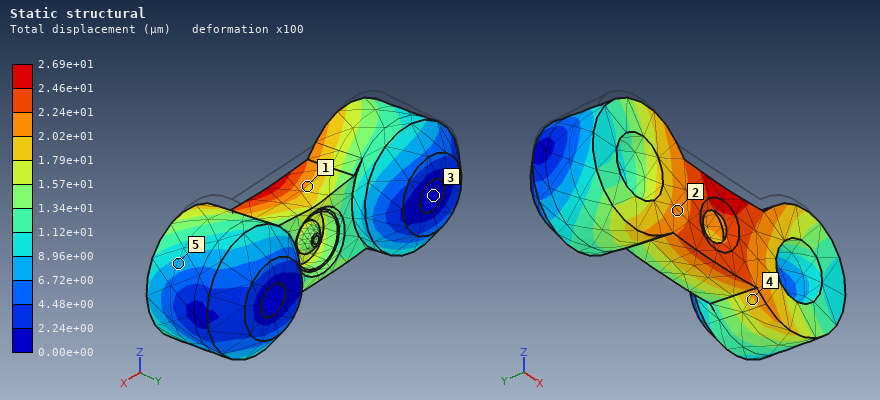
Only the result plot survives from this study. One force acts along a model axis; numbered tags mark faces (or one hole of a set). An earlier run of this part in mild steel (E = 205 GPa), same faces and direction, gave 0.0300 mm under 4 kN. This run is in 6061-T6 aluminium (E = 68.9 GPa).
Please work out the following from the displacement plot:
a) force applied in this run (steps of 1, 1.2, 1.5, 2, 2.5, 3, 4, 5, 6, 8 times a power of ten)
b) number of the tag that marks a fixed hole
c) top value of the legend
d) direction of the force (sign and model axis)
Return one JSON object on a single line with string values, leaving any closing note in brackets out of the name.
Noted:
{"force applied in this run": "1.2 kN", "number of the tag that marks a fixed hole": "3", "top value of the legend": "2.69e+01 µm", "direction of the force": "-Z"}
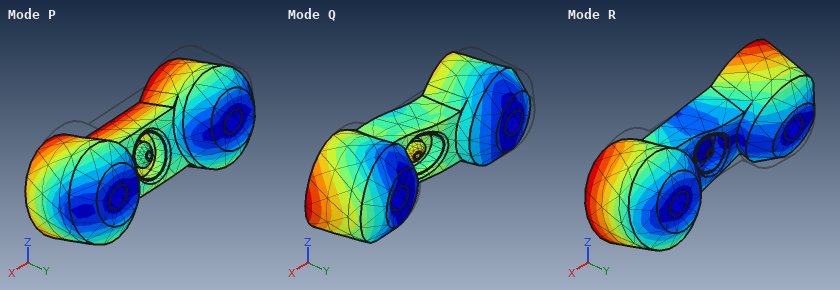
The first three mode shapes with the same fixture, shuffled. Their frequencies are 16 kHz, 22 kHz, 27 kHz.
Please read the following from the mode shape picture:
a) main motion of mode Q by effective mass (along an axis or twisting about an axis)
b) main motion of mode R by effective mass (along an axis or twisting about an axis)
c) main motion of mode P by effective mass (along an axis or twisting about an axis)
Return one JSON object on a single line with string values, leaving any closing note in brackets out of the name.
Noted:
{"main motion of mode Q by effective mass": "along X", "main motion of mode R by effective mass": "twisting about Y", "main motion of mode P by effective mass": "along Z"}
